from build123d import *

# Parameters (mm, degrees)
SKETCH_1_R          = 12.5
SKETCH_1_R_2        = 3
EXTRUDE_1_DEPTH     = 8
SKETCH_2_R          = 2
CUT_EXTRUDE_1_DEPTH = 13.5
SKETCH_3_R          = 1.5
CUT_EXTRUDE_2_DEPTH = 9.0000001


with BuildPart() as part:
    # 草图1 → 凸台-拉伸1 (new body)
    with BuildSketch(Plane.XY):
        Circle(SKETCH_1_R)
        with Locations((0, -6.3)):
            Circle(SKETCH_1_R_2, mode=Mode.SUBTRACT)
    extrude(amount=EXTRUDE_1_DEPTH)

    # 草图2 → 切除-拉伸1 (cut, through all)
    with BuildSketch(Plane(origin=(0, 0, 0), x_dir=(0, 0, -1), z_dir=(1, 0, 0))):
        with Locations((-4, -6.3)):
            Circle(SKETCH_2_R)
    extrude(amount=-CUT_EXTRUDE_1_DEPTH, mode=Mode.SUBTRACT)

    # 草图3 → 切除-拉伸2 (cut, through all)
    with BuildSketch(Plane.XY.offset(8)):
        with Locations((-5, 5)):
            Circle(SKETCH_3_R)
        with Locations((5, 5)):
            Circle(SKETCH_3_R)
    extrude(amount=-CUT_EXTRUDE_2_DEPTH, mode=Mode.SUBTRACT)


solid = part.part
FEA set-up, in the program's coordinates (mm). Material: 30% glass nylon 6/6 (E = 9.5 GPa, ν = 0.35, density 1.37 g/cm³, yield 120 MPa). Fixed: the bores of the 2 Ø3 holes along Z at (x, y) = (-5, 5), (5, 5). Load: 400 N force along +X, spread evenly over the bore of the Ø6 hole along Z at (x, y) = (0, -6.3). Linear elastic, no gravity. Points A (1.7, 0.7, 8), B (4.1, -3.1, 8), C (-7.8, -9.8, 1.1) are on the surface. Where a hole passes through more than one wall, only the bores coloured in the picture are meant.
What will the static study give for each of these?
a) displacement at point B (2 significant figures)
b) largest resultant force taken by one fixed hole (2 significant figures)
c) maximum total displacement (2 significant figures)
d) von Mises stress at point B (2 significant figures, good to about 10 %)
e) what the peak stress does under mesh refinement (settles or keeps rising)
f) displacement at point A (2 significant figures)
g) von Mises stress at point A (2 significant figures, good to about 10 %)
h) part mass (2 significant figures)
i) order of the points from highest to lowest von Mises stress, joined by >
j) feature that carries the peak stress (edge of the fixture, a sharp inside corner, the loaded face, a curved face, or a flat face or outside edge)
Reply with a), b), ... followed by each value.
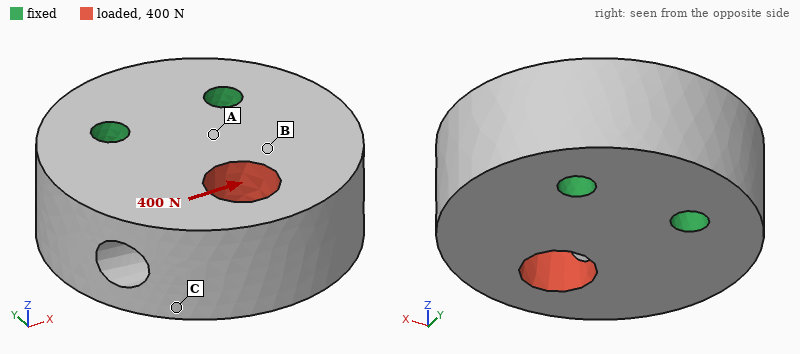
a) 10 µm
b) 400 N
c) 23 µm
d) 4.7 MPa
e) keeps rising
f) 4.4 µm
g) 8.1 MPa
h) 4.8 g
i) A > B > C
j) edge of the fixture
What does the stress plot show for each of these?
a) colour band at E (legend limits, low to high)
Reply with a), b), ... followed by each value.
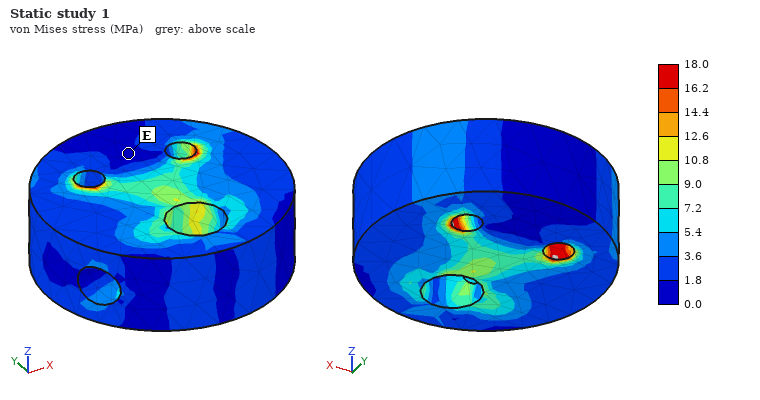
a) 0.0 to 1.8 MPa
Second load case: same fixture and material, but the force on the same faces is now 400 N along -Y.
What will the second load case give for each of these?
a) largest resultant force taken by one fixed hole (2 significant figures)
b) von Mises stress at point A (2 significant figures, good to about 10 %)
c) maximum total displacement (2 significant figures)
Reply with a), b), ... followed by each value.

a) 220 N
b) 2.8 MPa
c) 9.0 µm
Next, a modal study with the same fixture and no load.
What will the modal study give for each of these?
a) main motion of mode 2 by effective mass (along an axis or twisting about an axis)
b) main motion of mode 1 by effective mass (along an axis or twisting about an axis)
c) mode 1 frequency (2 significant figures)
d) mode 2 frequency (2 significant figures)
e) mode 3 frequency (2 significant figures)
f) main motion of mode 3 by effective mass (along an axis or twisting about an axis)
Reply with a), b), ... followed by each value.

a) along X
b) along Z
c) 12 kHz
d) 16 kHz
e) 19 kHz
f) twisting about Y
